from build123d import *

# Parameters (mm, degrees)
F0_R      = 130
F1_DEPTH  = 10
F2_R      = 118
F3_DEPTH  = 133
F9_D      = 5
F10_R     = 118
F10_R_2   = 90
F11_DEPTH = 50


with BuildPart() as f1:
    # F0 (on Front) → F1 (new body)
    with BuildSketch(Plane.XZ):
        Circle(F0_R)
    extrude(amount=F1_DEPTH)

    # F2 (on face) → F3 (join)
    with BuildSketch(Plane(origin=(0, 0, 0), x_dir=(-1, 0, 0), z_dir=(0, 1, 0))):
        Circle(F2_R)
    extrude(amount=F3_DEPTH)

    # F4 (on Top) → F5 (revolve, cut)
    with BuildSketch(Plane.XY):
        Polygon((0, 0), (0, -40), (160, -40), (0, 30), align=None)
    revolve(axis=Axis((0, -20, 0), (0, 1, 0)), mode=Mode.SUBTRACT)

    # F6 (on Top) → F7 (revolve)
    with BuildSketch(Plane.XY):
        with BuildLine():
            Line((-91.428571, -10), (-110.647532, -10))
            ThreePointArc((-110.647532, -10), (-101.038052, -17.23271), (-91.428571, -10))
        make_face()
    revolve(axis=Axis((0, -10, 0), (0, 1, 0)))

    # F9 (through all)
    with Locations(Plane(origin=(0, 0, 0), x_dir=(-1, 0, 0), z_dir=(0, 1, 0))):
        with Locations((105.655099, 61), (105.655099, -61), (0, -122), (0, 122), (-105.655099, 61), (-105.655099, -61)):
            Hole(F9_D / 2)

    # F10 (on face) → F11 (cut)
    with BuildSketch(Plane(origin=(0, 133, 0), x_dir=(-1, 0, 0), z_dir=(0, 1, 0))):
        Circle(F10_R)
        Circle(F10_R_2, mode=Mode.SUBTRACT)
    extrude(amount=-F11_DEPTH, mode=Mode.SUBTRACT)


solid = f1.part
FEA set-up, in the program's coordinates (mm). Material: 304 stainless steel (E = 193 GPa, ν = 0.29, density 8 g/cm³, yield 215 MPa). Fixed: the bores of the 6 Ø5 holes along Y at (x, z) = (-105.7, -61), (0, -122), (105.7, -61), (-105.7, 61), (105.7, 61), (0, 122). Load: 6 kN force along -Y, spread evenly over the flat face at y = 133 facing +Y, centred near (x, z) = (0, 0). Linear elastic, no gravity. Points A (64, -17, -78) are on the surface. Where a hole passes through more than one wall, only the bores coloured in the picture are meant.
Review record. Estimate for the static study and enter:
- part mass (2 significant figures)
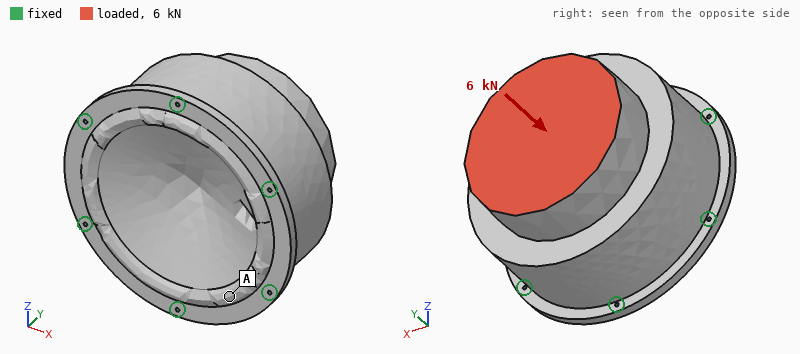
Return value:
41 kg
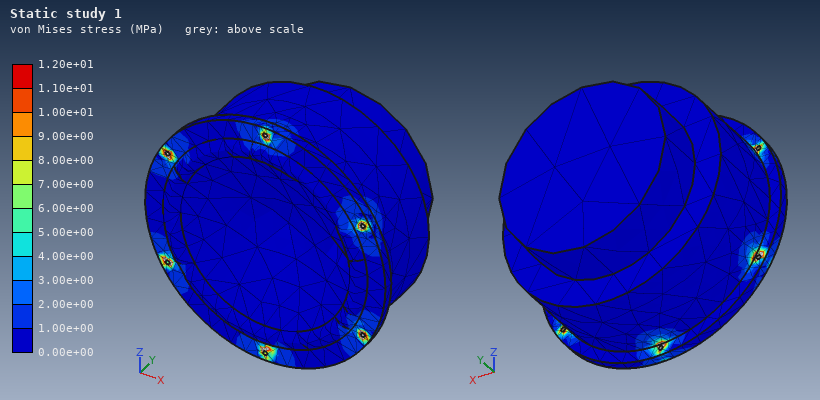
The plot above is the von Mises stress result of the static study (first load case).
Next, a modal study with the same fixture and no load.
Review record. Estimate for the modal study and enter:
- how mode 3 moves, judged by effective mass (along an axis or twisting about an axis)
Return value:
along Y
